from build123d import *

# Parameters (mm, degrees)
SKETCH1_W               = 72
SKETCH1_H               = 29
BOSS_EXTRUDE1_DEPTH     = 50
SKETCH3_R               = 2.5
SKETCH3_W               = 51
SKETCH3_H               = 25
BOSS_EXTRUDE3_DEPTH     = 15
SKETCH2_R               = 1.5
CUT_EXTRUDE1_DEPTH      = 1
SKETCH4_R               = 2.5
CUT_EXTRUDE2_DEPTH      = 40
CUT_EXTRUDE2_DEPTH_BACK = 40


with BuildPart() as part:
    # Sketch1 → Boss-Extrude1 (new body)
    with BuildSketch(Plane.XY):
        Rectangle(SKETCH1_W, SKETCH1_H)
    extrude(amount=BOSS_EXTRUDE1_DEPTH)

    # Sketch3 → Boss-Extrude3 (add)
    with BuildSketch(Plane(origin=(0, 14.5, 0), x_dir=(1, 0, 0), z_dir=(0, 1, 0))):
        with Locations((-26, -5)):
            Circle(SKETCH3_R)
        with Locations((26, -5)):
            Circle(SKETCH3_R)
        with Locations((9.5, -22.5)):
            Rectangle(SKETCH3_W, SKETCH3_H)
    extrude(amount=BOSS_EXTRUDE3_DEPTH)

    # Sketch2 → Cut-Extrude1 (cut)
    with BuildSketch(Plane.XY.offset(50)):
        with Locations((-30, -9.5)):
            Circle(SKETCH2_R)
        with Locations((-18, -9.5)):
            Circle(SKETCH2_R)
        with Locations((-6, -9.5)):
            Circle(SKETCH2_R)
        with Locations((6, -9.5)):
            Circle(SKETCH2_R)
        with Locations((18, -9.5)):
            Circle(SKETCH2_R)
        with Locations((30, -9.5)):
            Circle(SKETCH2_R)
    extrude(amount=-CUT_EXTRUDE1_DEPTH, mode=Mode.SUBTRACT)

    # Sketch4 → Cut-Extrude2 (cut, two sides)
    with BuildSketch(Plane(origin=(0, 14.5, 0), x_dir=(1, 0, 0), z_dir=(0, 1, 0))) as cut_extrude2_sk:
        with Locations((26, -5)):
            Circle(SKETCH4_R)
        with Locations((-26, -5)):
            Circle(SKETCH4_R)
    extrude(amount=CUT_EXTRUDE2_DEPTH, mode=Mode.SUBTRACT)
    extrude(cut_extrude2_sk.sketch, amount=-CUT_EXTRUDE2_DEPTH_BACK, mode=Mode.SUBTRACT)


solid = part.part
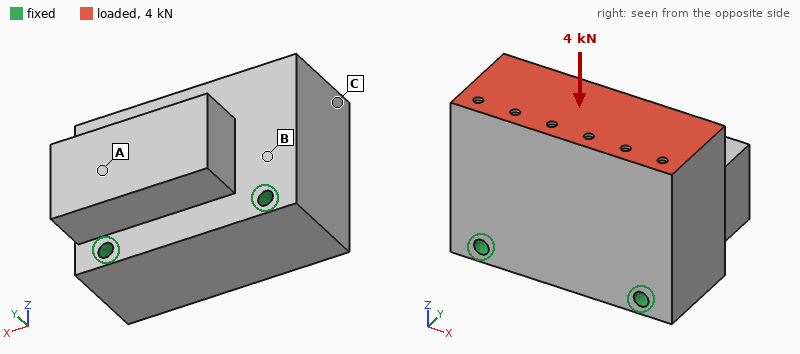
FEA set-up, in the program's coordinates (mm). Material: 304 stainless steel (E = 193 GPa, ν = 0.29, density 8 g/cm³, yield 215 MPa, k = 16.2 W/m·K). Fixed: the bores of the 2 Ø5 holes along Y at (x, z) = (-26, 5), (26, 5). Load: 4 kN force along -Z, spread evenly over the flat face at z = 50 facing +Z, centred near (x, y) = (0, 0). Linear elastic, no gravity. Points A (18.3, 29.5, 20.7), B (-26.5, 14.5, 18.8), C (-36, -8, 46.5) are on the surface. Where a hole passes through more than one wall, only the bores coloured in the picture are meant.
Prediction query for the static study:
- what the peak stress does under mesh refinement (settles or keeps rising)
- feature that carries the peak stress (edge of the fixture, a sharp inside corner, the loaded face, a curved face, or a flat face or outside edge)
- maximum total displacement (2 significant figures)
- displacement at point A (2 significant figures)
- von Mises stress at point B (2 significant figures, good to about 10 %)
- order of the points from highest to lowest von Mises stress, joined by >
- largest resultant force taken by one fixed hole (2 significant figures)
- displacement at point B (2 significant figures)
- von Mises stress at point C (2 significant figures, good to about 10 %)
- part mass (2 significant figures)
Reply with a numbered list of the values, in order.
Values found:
1. keeps rising
2. edge of the fixture
3. 0.69 µm
4. 0.38 µm
5. 3.0 MPa
6. B > C > A
7. 2.0 kN
8. 0.27 µm
9. 1.9 MPa
10. 980 g
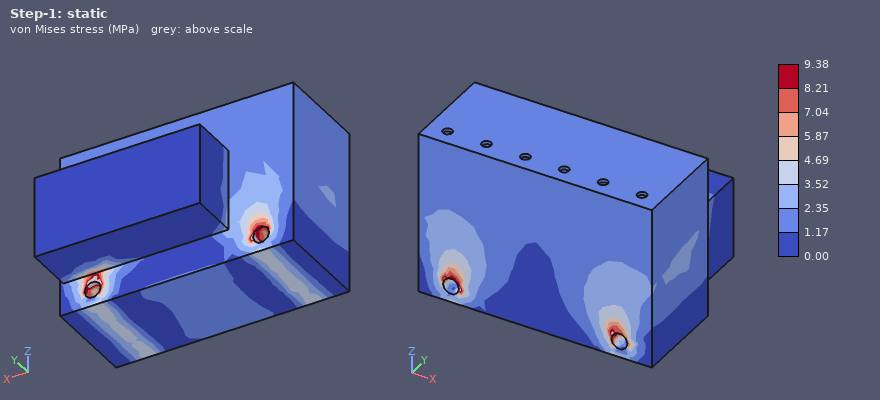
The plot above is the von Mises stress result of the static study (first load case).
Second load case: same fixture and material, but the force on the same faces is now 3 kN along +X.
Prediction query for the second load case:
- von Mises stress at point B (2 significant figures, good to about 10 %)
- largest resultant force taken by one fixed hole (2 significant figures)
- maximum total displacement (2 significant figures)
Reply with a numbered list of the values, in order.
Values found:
1. 3.7 MPa
2. 2.9 kN
3. 2.3 µm
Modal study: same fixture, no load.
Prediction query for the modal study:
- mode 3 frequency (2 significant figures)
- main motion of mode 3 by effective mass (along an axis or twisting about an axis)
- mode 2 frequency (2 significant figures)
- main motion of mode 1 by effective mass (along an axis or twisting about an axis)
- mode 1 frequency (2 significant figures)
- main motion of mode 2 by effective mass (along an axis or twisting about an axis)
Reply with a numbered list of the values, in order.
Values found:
1. 12 kHz
2. twisting about Z
3. 11 kHz
4. along Y
5. 6000 Hz
6. along X
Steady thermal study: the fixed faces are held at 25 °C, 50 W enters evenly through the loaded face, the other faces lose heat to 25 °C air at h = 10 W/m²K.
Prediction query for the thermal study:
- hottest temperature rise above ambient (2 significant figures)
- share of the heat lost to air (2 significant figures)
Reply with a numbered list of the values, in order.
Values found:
1. 71 K
2. 9.3 %
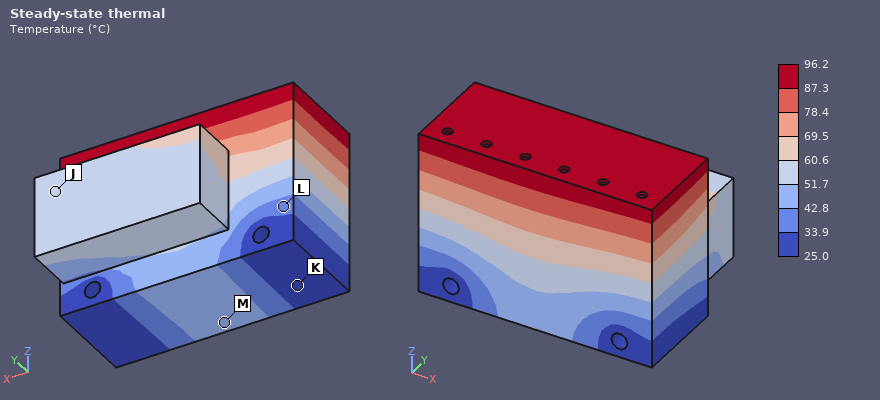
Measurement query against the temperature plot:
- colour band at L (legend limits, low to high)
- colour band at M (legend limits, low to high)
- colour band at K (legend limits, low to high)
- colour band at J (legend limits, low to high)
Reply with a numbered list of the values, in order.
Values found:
1. 33.9 to 42.8 °C
2. 42.8 to 51.7 °C
3. 25.0 to 33.9 °C
4. 51.7 to 60.6 °C
